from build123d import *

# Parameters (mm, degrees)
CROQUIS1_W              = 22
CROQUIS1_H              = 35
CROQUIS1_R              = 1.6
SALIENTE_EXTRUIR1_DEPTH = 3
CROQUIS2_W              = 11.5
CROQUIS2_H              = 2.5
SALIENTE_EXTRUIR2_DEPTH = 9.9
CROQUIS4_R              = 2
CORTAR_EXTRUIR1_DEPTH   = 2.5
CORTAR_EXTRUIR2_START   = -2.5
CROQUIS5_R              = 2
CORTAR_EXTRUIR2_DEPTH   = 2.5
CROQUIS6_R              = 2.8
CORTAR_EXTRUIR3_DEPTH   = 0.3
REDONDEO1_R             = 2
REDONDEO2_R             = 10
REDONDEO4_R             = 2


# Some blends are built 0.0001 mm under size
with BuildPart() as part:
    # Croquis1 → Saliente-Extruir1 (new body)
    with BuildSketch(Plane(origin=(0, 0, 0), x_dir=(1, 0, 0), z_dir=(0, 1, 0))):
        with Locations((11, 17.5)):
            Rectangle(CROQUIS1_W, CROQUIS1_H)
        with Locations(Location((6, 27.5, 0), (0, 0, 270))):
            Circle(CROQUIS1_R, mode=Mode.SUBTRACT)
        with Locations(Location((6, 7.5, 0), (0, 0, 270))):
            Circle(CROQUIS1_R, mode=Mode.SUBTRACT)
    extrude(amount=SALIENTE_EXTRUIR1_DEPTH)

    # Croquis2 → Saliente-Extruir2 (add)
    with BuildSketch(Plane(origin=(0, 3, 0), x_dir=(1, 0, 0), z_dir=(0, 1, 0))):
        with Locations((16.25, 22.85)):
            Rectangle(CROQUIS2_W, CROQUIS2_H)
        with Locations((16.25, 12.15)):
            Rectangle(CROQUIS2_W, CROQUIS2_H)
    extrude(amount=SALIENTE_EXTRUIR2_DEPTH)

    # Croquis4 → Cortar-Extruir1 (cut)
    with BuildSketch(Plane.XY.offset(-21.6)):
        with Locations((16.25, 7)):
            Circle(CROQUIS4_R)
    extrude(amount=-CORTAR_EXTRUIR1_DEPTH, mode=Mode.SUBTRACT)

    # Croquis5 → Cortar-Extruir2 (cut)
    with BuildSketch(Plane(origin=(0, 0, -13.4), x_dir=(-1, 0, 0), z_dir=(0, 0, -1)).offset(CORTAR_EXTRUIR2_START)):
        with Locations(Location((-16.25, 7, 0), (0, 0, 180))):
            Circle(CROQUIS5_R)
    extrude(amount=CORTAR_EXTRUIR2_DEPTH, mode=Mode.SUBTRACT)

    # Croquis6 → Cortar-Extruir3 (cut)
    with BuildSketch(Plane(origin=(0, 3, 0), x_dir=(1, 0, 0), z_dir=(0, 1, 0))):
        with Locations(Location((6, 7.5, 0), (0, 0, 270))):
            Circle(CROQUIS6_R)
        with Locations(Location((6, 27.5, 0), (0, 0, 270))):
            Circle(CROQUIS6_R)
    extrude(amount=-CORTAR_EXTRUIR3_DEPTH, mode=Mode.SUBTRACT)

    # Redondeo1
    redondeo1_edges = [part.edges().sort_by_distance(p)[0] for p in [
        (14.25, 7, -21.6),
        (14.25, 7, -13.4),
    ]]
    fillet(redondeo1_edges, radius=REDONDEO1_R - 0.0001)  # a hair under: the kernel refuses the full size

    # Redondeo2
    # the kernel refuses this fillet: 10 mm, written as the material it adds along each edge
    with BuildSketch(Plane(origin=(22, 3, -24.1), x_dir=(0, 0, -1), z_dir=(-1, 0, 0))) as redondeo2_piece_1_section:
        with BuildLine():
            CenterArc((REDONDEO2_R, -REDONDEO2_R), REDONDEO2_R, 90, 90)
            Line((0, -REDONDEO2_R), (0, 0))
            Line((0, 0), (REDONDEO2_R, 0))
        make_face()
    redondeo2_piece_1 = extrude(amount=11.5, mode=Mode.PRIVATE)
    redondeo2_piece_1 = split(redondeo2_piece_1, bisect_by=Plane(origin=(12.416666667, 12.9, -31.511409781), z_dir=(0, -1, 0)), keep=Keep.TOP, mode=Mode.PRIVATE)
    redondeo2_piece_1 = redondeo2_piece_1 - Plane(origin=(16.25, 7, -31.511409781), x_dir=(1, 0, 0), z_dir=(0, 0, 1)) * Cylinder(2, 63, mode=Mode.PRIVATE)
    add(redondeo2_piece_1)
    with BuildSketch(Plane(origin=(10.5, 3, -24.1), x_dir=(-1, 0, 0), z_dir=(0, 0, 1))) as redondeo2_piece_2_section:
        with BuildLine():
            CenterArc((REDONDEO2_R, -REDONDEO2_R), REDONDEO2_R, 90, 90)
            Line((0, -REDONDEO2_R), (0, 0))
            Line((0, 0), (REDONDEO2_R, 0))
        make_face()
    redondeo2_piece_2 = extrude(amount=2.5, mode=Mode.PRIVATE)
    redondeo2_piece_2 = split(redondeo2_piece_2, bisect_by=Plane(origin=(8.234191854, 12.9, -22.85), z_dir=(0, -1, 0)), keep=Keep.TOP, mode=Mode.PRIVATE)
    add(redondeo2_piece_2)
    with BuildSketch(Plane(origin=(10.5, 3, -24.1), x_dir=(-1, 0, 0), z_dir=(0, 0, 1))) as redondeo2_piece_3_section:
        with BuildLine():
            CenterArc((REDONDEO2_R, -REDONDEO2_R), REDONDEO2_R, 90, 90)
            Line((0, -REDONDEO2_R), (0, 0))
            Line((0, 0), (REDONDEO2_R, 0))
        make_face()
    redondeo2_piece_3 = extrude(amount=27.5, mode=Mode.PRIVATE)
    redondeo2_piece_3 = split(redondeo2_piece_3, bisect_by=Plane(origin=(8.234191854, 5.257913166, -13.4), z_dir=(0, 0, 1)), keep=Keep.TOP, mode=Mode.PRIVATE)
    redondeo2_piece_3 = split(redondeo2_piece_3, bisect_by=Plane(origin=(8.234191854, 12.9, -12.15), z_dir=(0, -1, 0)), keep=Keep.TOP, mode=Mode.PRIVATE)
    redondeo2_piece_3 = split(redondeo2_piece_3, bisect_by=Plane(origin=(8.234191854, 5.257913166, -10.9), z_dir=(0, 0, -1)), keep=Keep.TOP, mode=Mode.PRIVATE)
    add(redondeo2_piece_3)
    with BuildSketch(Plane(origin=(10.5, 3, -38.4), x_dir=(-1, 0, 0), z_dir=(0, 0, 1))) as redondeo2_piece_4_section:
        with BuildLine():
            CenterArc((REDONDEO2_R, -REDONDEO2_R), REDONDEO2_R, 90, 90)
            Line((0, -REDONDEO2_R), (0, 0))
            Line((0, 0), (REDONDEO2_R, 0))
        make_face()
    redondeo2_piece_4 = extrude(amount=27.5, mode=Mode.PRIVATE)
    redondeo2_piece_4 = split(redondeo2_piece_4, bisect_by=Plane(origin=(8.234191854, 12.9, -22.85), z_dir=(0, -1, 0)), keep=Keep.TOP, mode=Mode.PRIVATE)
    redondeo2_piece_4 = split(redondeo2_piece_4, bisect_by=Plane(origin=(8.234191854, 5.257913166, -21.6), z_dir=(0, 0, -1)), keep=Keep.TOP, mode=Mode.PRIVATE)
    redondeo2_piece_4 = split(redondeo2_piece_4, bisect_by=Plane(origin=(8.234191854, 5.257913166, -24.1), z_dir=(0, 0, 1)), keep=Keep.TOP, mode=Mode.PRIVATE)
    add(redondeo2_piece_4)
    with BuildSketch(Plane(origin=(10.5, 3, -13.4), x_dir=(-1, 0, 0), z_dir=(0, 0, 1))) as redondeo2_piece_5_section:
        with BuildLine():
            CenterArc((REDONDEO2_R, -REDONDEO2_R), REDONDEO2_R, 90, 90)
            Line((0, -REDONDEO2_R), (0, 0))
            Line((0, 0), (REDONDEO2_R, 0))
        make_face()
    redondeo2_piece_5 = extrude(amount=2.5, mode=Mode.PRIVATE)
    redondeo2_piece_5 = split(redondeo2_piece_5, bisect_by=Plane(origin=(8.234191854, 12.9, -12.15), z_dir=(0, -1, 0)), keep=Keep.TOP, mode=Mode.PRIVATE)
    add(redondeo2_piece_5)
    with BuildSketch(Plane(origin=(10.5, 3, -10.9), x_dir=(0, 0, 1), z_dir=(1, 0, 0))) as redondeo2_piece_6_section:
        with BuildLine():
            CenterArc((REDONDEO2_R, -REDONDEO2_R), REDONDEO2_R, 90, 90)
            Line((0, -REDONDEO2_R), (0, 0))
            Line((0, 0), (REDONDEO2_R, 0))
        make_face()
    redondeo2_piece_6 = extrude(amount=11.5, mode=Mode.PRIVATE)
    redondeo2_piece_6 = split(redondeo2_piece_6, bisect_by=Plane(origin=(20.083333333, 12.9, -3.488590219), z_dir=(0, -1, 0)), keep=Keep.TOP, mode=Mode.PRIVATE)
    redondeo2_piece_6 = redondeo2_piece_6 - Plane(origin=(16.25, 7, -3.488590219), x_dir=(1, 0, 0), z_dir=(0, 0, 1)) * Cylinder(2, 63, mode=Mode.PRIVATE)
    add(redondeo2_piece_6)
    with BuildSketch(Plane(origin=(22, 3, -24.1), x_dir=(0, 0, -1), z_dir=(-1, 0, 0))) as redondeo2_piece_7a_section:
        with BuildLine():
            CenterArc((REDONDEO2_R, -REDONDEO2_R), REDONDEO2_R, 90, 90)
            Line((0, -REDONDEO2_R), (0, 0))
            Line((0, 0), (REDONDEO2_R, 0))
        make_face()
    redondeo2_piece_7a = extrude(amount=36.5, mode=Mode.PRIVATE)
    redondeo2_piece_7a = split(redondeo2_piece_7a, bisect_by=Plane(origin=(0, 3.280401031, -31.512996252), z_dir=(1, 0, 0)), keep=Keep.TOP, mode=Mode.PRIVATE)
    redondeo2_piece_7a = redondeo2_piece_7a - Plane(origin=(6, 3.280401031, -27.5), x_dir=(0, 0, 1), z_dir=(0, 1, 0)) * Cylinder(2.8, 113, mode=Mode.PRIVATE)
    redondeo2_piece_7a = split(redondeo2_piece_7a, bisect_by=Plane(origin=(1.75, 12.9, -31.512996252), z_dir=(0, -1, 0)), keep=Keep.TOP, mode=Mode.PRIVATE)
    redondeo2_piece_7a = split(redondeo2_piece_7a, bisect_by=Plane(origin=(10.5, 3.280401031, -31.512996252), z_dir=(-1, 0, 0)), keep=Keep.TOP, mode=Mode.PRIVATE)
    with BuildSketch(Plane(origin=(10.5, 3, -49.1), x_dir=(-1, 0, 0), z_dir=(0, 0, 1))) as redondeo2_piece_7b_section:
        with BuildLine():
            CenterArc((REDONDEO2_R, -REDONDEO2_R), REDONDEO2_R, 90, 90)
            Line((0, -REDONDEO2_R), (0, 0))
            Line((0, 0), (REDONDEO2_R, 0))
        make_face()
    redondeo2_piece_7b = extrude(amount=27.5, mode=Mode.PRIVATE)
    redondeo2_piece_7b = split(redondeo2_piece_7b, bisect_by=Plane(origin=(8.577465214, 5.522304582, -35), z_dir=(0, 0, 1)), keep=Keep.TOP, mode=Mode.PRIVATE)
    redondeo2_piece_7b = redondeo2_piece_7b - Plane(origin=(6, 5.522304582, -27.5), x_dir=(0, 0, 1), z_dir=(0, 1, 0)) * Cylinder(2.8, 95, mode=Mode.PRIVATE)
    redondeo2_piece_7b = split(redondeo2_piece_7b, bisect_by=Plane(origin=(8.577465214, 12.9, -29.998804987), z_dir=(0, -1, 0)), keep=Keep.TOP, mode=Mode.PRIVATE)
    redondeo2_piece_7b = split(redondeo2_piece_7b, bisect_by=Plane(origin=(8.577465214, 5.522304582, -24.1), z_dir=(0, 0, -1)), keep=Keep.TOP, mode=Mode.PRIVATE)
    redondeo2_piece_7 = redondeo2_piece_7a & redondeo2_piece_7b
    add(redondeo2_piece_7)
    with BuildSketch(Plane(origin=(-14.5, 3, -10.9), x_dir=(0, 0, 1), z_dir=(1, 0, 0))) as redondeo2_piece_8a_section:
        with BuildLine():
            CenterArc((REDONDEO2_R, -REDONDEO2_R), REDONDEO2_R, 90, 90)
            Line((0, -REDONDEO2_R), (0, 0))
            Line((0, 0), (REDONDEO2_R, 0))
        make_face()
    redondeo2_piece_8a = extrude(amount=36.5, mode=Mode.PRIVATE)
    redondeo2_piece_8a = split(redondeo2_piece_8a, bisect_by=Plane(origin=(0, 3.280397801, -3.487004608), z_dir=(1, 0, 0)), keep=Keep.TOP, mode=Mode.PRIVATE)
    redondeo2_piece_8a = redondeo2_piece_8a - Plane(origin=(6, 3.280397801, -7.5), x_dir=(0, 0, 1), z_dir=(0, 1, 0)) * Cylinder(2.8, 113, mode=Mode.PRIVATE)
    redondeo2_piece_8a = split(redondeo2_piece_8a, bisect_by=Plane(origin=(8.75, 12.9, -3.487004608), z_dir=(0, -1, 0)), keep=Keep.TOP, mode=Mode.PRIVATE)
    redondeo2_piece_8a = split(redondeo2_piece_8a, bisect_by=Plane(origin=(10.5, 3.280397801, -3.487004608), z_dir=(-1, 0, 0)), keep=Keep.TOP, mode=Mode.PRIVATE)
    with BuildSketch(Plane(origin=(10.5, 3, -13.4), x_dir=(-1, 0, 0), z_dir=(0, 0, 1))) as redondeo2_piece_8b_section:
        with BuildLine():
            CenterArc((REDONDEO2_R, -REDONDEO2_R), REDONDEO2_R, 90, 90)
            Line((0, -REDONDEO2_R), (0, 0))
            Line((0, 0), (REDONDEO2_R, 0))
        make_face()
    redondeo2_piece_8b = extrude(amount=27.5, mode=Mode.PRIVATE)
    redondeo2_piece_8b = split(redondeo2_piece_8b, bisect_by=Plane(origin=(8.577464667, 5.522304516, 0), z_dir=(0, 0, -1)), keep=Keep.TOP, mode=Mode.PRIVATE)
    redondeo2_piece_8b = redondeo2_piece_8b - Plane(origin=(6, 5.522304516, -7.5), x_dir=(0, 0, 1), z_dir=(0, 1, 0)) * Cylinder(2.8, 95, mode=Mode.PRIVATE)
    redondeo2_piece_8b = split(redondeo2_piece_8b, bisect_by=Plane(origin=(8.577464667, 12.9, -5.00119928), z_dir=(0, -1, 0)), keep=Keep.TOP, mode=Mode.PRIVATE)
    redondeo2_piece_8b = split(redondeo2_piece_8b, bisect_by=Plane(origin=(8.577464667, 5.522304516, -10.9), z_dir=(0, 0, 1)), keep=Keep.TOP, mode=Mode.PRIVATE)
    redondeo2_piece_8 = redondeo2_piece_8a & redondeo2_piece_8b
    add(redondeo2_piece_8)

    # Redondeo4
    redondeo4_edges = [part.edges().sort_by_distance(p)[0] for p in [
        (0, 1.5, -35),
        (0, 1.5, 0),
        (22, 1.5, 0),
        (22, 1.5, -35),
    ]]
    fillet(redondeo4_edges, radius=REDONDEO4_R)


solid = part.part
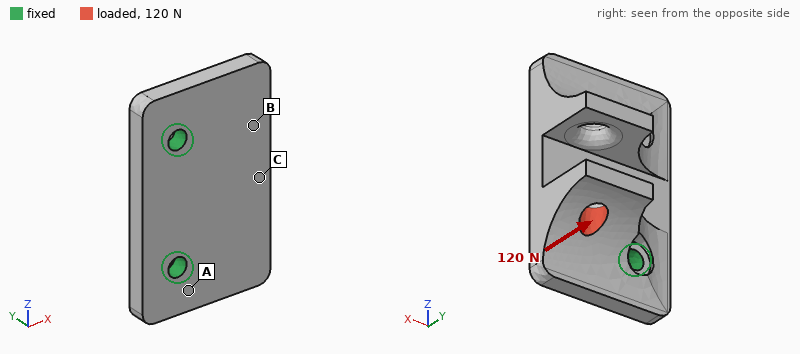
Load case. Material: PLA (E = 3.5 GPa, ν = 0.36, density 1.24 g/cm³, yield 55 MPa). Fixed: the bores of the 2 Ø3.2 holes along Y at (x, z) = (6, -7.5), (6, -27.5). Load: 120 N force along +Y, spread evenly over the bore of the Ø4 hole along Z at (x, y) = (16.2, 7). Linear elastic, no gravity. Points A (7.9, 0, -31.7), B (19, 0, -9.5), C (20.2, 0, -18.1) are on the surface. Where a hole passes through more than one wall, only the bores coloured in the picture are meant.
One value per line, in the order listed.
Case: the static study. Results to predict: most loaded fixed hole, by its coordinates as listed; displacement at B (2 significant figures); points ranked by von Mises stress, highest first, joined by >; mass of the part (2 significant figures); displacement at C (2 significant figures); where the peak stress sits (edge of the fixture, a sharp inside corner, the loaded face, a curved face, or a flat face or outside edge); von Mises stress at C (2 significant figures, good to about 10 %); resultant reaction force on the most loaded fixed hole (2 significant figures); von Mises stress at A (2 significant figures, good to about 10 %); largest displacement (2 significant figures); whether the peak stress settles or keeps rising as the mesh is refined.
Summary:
(6, -27.5)
0.13 mm
A > C > B
4.2 g
0.22 mm
edge of the fixture
6.4 MPa
100 N
11 MPa
0.36 mm
keeps rising
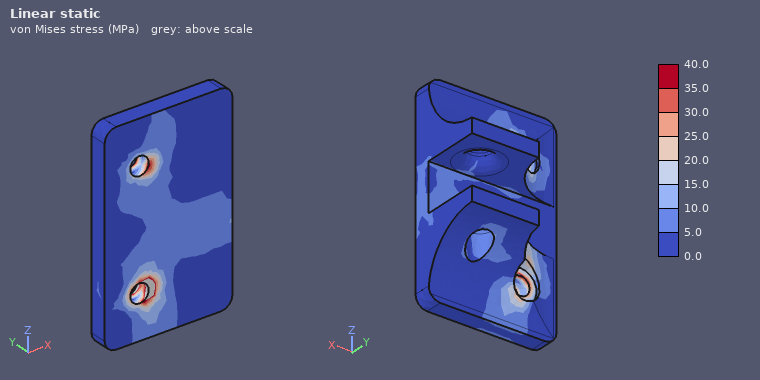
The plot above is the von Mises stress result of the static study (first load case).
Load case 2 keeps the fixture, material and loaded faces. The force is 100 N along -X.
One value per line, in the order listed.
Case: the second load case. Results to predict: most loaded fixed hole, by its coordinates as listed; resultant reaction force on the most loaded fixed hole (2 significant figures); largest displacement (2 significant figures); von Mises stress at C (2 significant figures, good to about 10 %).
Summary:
(6, -27.5)
88 N
0.17 mm
3.1 MPa
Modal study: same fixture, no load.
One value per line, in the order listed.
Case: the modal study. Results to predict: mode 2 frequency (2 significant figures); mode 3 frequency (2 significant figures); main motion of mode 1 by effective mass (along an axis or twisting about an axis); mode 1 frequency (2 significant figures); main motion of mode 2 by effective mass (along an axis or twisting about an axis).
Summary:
4400 Hz
5800 Hz
along Y
2500 Hz
twisting about X
